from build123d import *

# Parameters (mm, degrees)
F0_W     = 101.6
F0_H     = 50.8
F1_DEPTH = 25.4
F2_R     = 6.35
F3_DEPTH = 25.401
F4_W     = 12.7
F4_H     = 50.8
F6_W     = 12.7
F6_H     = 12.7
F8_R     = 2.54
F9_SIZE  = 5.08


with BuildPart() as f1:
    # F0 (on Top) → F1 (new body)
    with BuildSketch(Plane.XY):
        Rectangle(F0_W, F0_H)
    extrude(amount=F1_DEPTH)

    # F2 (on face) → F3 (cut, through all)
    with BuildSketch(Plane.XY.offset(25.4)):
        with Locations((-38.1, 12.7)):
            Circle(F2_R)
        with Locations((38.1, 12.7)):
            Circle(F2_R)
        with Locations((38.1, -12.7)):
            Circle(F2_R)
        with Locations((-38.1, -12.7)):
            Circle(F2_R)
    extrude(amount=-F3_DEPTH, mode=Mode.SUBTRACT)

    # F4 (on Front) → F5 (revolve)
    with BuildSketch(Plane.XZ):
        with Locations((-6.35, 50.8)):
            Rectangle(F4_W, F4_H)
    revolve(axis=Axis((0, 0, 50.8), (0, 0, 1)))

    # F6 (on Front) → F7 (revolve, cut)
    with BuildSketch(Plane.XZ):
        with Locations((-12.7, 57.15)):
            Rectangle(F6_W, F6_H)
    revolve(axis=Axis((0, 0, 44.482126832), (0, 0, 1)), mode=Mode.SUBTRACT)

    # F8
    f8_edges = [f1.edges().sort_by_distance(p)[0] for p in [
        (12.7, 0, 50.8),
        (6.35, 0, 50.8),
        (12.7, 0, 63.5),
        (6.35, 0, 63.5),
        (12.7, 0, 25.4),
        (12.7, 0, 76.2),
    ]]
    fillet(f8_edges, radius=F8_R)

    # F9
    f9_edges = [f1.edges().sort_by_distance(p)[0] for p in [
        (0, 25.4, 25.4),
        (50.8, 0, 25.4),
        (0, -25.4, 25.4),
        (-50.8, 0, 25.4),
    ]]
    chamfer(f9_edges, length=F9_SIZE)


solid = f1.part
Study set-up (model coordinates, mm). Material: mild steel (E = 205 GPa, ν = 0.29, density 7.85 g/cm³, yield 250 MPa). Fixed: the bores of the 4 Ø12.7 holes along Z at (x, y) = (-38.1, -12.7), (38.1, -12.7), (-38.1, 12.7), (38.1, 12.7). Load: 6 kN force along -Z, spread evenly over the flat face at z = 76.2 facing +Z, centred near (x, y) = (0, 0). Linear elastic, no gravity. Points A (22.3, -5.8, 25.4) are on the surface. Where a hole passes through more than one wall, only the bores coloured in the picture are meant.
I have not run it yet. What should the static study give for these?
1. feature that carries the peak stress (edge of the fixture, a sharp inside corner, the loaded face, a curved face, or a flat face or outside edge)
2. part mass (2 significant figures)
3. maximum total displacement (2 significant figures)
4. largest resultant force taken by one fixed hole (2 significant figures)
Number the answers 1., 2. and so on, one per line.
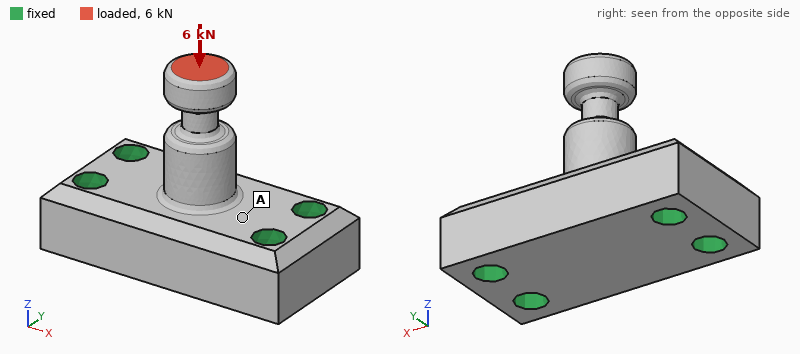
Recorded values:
1. a curved face
2. 1.1 kg
3. 7.8 µm
4. 1.5 kN
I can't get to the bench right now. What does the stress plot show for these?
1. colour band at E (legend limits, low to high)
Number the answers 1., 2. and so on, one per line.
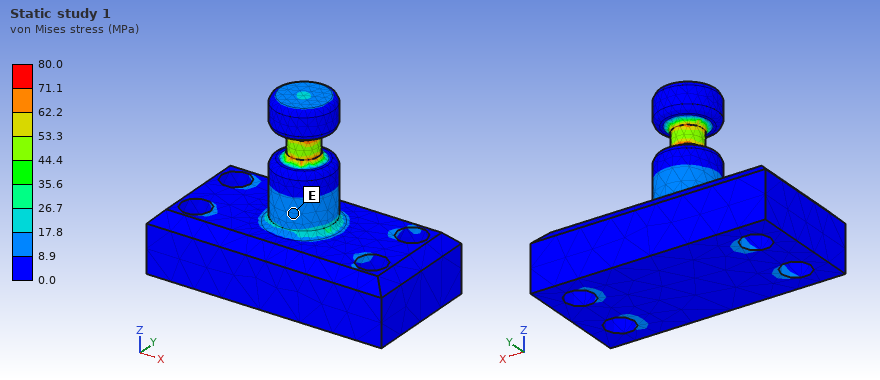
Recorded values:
1. 8.9 to 17.8 MPa
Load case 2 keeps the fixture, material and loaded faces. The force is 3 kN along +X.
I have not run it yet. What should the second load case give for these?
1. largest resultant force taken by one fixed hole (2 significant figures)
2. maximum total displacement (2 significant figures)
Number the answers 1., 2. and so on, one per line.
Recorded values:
1. 1.9 kN
2. 0.12 mm
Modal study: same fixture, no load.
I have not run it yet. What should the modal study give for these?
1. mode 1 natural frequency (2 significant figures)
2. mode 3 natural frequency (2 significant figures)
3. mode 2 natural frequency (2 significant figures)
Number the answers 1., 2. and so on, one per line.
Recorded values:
1. 4300 Hz
2. 9100 Hz
3. 4500 Hz
